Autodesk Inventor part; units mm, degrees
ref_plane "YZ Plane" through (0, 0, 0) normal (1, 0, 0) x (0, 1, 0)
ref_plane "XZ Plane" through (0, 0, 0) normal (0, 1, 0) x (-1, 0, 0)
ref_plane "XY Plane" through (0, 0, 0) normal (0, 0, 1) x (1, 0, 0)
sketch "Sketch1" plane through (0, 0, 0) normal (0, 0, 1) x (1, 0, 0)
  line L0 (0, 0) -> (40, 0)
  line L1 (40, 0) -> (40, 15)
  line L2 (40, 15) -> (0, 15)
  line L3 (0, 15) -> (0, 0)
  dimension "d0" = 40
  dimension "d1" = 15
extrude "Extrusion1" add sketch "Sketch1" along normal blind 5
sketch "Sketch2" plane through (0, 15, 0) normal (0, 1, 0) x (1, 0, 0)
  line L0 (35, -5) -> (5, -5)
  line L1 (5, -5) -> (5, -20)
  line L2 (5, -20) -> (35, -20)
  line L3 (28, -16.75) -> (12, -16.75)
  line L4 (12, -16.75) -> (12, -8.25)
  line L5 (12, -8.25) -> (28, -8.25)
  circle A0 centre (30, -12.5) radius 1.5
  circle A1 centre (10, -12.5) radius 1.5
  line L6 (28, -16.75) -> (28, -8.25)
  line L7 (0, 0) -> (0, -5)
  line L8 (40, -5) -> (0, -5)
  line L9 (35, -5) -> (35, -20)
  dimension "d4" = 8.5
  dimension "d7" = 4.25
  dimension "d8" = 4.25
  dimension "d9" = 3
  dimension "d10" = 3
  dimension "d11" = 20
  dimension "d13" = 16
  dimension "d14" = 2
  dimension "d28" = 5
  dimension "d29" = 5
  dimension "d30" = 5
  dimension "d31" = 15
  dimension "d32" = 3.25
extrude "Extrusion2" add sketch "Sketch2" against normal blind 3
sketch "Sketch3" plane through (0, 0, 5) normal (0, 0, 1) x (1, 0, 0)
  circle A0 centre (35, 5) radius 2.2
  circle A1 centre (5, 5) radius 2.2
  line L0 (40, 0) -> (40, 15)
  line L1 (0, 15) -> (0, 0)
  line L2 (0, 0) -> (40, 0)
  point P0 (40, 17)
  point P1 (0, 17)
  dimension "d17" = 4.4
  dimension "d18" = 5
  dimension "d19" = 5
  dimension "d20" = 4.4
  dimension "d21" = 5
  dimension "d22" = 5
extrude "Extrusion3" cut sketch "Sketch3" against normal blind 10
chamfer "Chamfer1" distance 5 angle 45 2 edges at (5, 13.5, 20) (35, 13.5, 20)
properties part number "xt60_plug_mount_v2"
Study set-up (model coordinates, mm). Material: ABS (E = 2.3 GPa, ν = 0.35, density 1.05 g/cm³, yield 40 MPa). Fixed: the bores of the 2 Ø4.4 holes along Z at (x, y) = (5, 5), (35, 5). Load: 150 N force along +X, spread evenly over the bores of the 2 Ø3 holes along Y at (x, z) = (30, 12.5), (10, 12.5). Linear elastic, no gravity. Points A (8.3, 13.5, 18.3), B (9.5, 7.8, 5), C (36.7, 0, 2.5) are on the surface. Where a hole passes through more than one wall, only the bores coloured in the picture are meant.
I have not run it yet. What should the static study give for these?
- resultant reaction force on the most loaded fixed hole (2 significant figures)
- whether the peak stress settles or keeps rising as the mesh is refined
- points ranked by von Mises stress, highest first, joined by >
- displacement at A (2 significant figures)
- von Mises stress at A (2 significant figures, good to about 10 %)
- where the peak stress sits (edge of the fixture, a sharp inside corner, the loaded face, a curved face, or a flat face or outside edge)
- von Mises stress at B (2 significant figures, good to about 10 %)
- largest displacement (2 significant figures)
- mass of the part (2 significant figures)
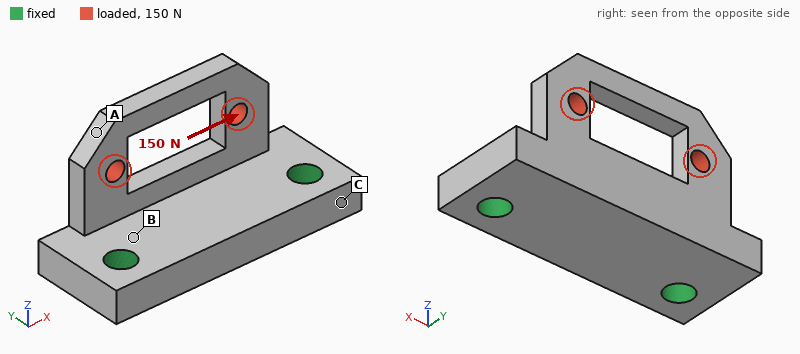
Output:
96 N
keeps rising
A > B > C
0.18 mm
5.8 MPa
a sharp inside corner
3.9 MPa
0.20 mm
3.9 g
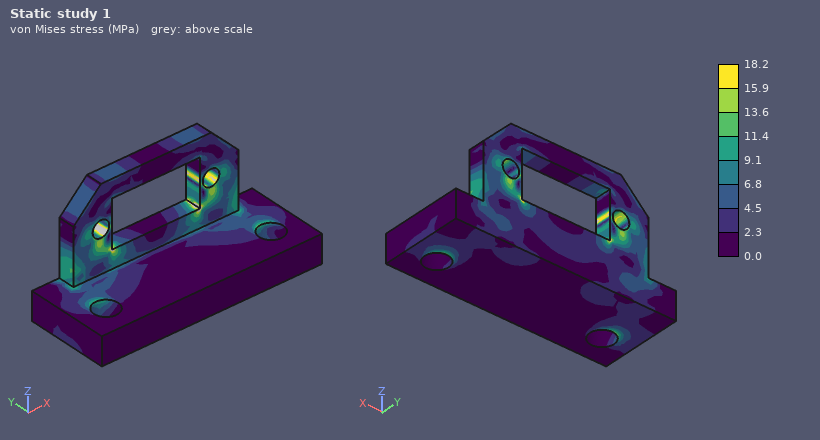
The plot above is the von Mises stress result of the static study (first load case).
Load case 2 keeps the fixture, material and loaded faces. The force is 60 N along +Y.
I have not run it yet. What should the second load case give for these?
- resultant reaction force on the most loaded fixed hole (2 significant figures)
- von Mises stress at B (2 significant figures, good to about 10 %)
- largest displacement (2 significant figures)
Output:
32 N
4.1 MPa
0.51 mm
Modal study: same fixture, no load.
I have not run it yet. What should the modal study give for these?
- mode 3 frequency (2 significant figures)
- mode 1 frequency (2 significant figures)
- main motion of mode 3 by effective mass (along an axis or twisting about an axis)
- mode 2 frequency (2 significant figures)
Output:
5400 Hz
2100 Hz
along X
3800 Hz
